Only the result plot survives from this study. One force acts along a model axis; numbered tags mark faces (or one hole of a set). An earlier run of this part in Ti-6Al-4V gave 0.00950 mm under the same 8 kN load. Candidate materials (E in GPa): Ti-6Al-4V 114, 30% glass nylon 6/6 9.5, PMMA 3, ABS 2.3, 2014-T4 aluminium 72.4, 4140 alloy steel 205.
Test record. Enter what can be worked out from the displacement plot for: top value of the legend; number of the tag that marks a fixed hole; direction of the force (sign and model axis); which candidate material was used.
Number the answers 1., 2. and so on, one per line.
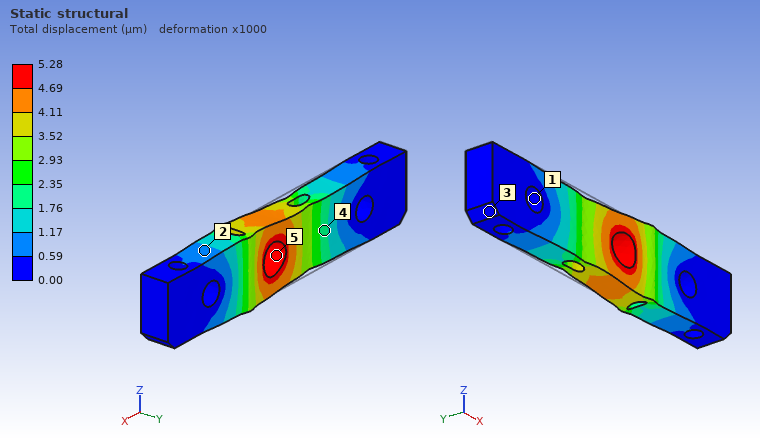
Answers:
1. 5.28 µm
2. 1
3. +X
4. 4140 alloy steel
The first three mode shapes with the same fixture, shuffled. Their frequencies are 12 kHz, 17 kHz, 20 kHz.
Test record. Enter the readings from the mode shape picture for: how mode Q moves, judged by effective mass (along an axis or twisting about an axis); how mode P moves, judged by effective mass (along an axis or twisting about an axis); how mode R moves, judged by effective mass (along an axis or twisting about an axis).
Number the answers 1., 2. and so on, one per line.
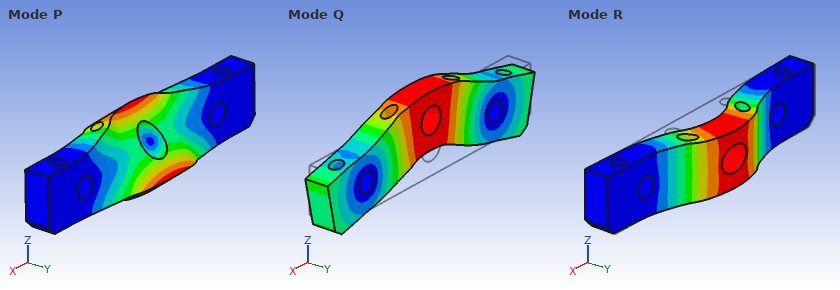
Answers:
1. along Z
2. twisting about X
3. along Y
